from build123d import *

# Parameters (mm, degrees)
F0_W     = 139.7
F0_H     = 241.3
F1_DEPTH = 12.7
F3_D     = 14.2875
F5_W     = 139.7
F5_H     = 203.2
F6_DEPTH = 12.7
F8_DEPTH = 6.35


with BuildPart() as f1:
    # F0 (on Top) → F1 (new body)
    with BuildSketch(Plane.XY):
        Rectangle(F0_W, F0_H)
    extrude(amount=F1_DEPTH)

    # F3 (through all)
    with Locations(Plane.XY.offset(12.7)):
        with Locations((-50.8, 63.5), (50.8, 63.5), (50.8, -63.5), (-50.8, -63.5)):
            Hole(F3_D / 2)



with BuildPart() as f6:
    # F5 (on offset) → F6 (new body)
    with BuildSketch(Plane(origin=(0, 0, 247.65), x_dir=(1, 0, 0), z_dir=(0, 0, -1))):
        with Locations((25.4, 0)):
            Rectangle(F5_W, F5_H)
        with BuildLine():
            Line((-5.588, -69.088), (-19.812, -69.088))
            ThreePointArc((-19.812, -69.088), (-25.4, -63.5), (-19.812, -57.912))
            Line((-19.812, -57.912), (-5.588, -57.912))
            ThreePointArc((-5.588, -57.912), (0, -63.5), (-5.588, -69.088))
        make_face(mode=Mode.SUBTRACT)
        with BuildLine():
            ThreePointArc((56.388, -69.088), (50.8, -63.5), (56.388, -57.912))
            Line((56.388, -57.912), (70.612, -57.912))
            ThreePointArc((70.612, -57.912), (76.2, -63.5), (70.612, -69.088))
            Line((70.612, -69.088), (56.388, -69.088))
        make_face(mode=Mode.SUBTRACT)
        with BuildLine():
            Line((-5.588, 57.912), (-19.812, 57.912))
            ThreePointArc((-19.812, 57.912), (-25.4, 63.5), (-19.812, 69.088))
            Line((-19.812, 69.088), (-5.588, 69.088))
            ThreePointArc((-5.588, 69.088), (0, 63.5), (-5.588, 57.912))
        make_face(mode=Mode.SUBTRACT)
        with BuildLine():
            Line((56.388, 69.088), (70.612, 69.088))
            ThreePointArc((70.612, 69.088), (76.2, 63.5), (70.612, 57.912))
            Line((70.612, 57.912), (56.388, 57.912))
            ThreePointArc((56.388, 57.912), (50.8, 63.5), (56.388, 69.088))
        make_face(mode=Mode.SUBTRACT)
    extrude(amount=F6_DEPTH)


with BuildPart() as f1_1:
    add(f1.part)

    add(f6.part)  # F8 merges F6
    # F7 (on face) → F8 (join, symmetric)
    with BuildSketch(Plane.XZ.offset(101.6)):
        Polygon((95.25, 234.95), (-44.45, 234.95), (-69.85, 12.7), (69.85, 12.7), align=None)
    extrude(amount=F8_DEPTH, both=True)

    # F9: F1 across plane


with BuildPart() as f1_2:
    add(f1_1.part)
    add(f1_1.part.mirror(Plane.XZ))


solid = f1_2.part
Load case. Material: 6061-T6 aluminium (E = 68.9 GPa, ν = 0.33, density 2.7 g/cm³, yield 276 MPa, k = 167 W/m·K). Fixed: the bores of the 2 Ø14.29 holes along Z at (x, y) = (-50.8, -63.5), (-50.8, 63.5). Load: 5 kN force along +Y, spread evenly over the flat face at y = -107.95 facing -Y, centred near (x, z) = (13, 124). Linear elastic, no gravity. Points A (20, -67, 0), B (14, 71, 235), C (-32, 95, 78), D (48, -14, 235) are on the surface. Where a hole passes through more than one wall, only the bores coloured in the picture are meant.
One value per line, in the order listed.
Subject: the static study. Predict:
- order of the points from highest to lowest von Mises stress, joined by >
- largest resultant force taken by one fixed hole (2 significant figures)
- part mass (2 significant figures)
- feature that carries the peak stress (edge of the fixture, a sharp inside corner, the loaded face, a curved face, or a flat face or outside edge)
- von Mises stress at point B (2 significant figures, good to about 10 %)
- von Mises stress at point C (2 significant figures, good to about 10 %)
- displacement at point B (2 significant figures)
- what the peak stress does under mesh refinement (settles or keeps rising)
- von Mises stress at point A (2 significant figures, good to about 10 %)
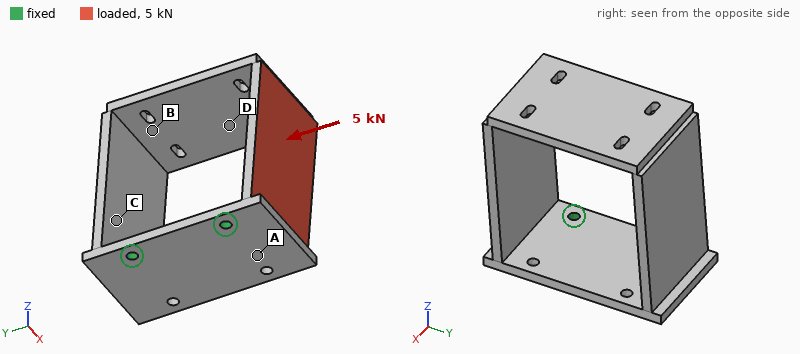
A > B > C > D
4.4 kN
4.2 kg
edge of the fixture
31 MPa
19 MPa
2.0 mm
keeps rising
43 MPa
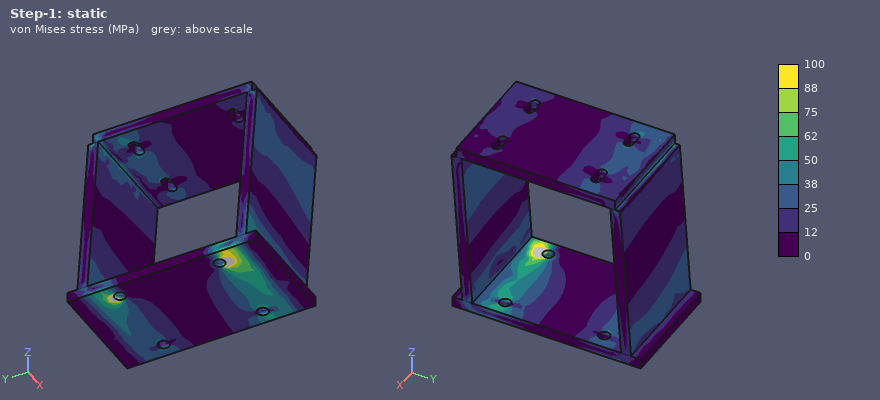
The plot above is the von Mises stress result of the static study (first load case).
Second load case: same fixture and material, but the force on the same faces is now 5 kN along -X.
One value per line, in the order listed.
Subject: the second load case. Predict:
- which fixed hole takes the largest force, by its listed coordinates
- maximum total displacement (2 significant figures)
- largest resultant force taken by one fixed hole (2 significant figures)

(-50.8, -63.5)
2.4 mm
6.5 kN
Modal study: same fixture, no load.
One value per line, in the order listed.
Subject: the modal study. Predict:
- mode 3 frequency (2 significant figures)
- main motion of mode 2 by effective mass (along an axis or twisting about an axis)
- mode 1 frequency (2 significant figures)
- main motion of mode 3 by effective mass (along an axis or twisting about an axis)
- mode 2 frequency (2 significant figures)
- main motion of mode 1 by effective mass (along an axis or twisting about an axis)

320 Hz
along X
140 Hz
twisting about Z
140 Hz
along Y
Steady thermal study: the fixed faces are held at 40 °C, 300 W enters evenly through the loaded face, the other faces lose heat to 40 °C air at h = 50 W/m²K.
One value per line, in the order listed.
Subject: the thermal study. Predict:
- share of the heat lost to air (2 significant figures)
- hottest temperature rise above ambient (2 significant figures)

68 %
55 K
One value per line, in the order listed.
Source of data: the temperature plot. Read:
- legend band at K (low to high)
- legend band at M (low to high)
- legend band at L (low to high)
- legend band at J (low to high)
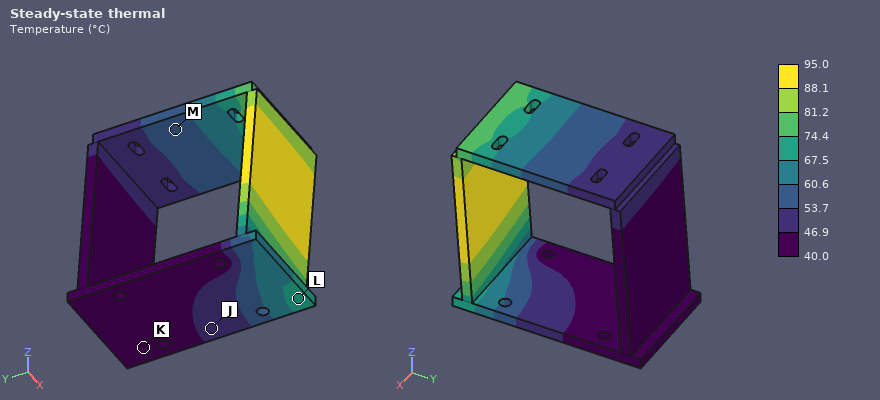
40.0 to 46.9 °C
53.7 to 60.6 °C
67.5 to 74.4 °C
46.9 to 53.7 °C
